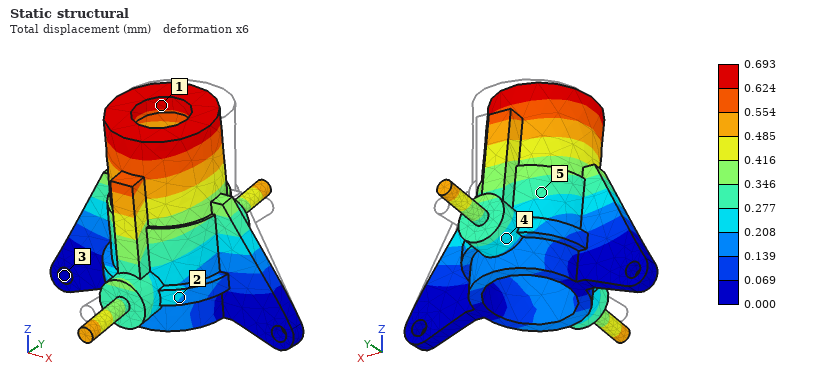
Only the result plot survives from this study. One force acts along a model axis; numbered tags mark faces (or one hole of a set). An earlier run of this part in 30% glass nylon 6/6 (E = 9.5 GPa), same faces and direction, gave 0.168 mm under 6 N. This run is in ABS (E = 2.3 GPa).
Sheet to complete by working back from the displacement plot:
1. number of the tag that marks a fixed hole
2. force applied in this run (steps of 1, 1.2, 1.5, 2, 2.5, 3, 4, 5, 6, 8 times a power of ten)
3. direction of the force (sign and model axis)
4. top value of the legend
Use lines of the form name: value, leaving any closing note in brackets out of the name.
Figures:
number of the tag that marks a fixed hole: 3
force applied in this run: 6 N
direction of the force: -Y
top value of the legend: 0.693 mm
